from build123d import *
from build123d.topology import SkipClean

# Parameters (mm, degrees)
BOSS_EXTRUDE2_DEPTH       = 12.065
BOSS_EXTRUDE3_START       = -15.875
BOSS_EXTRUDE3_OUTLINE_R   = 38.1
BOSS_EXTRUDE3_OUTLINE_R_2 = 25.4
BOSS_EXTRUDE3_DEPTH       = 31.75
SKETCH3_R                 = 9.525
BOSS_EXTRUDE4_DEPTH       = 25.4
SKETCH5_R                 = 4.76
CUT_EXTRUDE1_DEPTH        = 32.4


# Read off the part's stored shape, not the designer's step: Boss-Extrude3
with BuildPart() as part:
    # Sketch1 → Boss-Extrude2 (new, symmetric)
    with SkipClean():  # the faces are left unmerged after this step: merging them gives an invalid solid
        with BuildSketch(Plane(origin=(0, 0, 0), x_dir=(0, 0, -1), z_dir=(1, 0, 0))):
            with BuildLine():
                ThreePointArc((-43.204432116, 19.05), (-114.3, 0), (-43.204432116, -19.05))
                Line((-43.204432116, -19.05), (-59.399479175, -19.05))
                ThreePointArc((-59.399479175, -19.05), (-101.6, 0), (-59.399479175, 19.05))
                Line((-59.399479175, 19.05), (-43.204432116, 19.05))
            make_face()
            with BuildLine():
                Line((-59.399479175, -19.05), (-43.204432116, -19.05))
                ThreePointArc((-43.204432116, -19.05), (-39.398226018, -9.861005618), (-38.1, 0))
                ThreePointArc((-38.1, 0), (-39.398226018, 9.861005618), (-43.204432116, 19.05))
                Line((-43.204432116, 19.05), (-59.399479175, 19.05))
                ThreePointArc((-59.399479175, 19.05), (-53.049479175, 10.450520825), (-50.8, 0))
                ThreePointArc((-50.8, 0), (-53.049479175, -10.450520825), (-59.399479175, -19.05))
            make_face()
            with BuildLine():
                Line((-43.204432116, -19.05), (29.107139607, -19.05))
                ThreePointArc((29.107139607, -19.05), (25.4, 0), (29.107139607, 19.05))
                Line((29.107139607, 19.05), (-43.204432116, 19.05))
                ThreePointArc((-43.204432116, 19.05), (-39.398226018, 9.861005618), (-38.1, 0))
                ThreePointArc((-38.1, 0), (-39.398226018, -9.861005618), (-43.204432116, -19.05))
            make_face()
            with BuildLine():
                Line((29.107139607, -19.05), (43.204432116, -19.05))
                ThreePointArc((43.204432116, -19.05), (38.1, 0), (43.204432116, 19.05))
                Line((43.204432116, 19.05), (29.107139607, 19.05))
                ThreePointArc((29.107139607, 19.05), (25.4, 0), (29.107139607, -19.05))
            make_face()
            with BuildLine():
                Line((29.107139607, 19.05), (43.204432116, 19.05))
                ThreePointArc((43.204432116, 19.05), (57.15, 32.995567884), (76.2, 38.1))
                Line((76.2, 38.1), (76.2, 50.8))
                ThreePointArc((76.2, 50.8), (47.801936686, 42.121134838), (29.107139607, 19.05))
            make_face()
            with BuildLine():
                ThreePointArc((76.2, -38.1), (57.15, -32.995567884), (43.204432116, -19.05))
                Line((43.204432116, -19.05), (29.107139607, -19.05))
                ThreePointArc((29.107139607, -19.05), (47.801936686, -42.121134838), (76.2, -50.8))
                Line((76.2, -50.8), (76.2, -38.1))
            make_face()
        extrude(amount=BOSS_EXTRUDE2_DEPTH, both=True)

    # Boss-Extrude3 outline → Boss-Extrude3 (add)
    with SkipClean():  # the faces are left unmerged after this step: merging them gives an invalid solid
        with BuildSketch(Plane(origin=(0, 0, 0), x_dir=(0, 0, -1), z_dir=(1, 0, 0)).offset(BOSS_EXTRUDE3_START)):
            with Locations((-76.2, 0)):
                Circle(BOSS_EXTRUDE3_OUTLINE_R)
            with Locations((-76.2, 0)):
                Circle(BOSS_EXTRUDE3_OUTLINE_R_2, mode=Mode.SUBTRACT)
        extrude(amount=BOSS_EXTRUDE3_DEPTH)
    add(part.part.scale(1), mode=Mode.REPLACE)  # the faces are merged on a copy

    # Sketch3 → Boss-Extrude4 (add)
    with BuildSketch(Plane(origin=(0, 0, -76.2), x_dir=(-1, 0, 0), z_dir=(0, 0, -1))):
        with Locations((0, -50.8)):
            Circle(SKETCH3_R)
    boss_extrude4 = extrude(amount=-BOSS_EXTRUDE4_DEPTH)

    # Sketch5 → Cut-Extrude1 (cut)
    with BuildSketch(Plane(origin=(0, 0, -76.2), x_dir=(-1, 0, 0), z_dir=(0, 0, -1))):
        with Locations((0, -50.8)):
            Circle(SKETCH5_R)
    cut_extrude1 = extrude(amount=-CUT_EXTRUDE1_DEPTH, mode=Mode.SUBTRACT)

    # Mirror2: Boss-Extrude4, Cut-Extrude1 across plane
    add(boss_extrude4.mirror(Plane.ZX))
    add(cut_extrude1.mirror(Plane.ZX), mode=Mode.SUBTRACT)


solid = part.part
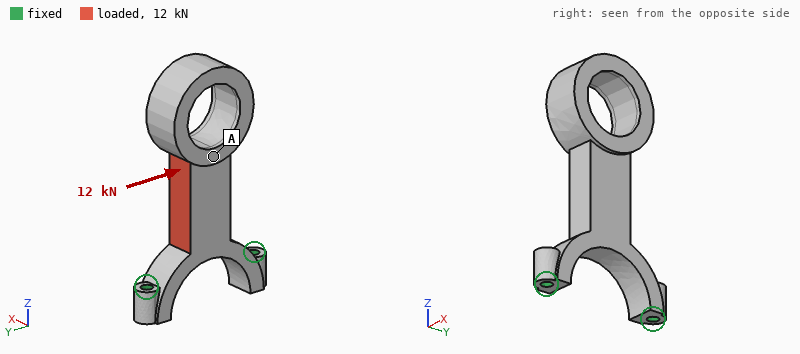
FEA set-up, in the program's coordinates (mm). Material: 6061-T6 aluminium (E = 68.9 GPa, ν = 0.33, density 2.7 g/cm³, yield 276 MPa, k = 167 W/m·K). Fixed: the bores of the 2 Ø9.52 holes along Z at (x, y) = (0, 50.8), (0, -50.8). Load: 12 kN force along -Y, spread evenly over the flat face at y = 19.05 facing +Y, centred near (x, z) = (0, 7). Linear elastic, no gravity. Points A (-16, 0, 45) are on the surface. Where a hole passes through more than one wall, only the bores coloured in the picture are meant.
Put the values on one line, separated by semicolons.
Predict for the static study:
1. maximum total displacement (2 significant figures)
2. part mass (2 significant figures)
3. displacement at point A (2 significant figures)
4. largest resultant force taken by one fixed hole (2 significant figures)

0.59 mm; 510 g; 0.30 mm; 12 kN
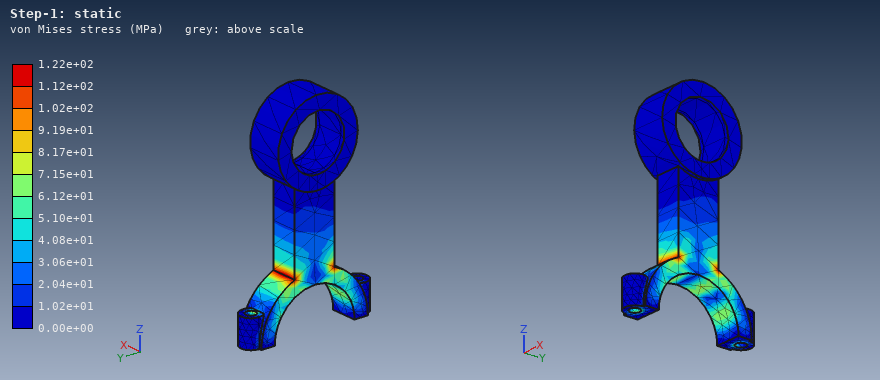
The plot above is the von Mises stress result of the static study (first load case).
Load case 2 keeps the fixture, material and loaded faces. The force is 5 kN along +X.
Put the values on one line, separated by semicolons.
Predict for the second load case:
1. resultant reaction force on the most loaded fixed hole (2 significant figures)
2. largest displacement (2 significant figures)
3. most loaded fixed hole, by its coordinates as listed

3.7 kN; 1.8 mm; (0, 50.8)
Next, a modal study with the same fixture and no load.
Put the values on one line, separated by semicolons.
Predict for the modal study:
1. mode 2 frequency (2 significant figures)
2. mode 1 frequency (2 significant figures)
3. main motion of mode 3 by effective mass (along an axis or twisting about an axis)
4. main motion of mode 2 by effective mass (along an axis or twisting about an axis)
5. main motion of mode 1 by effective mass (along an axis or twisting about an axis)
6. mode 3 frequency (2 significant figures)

810 Hz; 380 Hz; twisting about Z; along Y; along X; 2100 Hz
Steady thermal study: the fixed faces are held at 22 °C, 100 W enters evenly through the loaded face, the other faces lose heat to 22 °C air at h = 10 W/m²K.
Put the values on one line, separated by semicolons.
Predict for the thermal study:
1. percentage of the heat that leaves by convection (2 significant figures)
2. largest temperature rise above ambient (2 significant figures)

14 %; 60 K
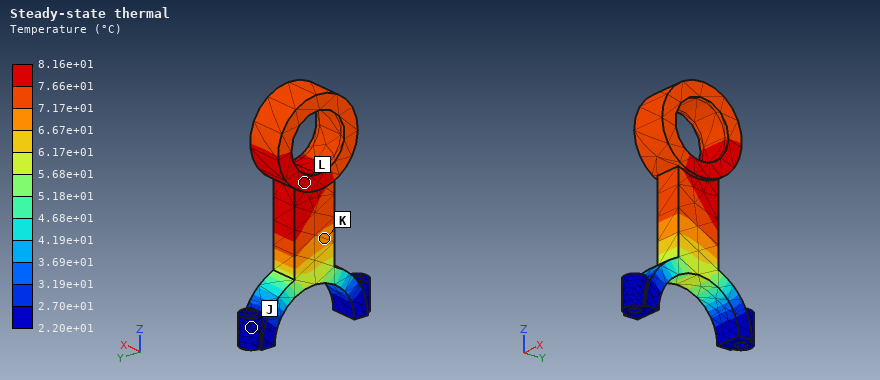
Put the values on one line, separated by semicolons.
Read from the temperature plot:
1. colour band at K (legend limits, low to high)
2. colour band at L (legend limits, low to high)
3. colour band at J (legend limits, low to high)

6.67e+01 to 7.17e+01 °C; 7.66e+01 to 8.16e+01 °C; 2.20e+01 to 2.70e+01 °C
